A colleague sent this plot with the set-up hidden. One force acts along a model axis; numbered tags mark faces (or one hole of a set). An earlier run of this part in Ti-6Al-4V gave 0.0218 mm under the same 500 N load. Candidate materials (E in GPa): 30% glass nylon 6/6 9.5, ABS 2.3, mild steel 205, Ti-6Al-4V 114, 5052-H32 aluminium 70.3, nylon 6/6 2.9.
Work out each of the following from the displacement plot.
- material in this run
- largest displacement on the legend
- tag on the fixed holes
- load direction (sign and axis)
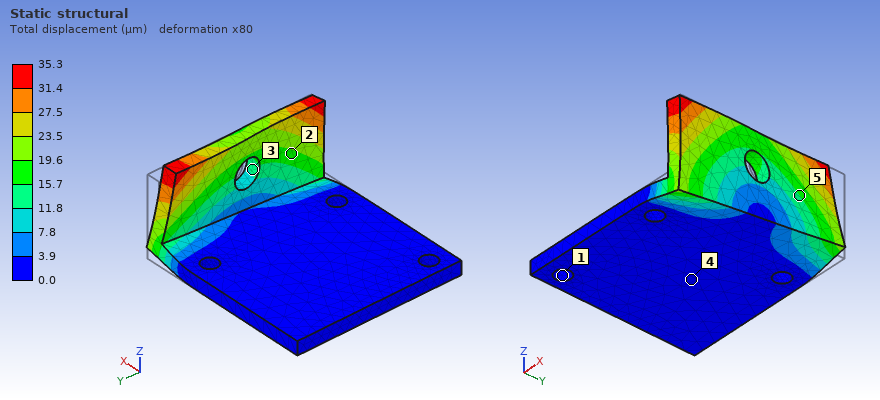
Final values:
5052-H32 aluminium
35.3 µm
1
-Y
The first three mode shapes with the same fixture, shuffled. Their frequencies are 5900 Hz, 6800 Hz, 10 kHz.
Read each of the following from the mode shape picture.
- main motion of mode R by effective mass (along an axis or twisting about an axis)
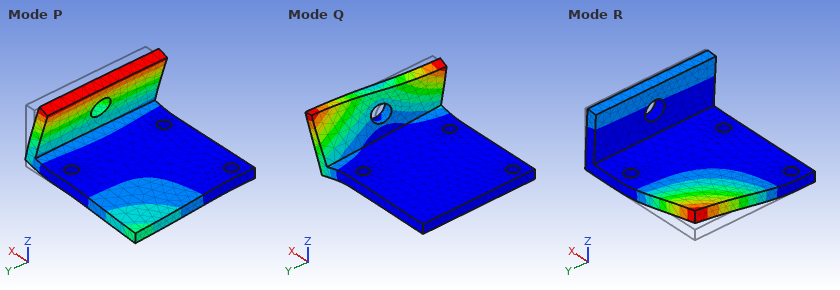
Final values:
along Z
